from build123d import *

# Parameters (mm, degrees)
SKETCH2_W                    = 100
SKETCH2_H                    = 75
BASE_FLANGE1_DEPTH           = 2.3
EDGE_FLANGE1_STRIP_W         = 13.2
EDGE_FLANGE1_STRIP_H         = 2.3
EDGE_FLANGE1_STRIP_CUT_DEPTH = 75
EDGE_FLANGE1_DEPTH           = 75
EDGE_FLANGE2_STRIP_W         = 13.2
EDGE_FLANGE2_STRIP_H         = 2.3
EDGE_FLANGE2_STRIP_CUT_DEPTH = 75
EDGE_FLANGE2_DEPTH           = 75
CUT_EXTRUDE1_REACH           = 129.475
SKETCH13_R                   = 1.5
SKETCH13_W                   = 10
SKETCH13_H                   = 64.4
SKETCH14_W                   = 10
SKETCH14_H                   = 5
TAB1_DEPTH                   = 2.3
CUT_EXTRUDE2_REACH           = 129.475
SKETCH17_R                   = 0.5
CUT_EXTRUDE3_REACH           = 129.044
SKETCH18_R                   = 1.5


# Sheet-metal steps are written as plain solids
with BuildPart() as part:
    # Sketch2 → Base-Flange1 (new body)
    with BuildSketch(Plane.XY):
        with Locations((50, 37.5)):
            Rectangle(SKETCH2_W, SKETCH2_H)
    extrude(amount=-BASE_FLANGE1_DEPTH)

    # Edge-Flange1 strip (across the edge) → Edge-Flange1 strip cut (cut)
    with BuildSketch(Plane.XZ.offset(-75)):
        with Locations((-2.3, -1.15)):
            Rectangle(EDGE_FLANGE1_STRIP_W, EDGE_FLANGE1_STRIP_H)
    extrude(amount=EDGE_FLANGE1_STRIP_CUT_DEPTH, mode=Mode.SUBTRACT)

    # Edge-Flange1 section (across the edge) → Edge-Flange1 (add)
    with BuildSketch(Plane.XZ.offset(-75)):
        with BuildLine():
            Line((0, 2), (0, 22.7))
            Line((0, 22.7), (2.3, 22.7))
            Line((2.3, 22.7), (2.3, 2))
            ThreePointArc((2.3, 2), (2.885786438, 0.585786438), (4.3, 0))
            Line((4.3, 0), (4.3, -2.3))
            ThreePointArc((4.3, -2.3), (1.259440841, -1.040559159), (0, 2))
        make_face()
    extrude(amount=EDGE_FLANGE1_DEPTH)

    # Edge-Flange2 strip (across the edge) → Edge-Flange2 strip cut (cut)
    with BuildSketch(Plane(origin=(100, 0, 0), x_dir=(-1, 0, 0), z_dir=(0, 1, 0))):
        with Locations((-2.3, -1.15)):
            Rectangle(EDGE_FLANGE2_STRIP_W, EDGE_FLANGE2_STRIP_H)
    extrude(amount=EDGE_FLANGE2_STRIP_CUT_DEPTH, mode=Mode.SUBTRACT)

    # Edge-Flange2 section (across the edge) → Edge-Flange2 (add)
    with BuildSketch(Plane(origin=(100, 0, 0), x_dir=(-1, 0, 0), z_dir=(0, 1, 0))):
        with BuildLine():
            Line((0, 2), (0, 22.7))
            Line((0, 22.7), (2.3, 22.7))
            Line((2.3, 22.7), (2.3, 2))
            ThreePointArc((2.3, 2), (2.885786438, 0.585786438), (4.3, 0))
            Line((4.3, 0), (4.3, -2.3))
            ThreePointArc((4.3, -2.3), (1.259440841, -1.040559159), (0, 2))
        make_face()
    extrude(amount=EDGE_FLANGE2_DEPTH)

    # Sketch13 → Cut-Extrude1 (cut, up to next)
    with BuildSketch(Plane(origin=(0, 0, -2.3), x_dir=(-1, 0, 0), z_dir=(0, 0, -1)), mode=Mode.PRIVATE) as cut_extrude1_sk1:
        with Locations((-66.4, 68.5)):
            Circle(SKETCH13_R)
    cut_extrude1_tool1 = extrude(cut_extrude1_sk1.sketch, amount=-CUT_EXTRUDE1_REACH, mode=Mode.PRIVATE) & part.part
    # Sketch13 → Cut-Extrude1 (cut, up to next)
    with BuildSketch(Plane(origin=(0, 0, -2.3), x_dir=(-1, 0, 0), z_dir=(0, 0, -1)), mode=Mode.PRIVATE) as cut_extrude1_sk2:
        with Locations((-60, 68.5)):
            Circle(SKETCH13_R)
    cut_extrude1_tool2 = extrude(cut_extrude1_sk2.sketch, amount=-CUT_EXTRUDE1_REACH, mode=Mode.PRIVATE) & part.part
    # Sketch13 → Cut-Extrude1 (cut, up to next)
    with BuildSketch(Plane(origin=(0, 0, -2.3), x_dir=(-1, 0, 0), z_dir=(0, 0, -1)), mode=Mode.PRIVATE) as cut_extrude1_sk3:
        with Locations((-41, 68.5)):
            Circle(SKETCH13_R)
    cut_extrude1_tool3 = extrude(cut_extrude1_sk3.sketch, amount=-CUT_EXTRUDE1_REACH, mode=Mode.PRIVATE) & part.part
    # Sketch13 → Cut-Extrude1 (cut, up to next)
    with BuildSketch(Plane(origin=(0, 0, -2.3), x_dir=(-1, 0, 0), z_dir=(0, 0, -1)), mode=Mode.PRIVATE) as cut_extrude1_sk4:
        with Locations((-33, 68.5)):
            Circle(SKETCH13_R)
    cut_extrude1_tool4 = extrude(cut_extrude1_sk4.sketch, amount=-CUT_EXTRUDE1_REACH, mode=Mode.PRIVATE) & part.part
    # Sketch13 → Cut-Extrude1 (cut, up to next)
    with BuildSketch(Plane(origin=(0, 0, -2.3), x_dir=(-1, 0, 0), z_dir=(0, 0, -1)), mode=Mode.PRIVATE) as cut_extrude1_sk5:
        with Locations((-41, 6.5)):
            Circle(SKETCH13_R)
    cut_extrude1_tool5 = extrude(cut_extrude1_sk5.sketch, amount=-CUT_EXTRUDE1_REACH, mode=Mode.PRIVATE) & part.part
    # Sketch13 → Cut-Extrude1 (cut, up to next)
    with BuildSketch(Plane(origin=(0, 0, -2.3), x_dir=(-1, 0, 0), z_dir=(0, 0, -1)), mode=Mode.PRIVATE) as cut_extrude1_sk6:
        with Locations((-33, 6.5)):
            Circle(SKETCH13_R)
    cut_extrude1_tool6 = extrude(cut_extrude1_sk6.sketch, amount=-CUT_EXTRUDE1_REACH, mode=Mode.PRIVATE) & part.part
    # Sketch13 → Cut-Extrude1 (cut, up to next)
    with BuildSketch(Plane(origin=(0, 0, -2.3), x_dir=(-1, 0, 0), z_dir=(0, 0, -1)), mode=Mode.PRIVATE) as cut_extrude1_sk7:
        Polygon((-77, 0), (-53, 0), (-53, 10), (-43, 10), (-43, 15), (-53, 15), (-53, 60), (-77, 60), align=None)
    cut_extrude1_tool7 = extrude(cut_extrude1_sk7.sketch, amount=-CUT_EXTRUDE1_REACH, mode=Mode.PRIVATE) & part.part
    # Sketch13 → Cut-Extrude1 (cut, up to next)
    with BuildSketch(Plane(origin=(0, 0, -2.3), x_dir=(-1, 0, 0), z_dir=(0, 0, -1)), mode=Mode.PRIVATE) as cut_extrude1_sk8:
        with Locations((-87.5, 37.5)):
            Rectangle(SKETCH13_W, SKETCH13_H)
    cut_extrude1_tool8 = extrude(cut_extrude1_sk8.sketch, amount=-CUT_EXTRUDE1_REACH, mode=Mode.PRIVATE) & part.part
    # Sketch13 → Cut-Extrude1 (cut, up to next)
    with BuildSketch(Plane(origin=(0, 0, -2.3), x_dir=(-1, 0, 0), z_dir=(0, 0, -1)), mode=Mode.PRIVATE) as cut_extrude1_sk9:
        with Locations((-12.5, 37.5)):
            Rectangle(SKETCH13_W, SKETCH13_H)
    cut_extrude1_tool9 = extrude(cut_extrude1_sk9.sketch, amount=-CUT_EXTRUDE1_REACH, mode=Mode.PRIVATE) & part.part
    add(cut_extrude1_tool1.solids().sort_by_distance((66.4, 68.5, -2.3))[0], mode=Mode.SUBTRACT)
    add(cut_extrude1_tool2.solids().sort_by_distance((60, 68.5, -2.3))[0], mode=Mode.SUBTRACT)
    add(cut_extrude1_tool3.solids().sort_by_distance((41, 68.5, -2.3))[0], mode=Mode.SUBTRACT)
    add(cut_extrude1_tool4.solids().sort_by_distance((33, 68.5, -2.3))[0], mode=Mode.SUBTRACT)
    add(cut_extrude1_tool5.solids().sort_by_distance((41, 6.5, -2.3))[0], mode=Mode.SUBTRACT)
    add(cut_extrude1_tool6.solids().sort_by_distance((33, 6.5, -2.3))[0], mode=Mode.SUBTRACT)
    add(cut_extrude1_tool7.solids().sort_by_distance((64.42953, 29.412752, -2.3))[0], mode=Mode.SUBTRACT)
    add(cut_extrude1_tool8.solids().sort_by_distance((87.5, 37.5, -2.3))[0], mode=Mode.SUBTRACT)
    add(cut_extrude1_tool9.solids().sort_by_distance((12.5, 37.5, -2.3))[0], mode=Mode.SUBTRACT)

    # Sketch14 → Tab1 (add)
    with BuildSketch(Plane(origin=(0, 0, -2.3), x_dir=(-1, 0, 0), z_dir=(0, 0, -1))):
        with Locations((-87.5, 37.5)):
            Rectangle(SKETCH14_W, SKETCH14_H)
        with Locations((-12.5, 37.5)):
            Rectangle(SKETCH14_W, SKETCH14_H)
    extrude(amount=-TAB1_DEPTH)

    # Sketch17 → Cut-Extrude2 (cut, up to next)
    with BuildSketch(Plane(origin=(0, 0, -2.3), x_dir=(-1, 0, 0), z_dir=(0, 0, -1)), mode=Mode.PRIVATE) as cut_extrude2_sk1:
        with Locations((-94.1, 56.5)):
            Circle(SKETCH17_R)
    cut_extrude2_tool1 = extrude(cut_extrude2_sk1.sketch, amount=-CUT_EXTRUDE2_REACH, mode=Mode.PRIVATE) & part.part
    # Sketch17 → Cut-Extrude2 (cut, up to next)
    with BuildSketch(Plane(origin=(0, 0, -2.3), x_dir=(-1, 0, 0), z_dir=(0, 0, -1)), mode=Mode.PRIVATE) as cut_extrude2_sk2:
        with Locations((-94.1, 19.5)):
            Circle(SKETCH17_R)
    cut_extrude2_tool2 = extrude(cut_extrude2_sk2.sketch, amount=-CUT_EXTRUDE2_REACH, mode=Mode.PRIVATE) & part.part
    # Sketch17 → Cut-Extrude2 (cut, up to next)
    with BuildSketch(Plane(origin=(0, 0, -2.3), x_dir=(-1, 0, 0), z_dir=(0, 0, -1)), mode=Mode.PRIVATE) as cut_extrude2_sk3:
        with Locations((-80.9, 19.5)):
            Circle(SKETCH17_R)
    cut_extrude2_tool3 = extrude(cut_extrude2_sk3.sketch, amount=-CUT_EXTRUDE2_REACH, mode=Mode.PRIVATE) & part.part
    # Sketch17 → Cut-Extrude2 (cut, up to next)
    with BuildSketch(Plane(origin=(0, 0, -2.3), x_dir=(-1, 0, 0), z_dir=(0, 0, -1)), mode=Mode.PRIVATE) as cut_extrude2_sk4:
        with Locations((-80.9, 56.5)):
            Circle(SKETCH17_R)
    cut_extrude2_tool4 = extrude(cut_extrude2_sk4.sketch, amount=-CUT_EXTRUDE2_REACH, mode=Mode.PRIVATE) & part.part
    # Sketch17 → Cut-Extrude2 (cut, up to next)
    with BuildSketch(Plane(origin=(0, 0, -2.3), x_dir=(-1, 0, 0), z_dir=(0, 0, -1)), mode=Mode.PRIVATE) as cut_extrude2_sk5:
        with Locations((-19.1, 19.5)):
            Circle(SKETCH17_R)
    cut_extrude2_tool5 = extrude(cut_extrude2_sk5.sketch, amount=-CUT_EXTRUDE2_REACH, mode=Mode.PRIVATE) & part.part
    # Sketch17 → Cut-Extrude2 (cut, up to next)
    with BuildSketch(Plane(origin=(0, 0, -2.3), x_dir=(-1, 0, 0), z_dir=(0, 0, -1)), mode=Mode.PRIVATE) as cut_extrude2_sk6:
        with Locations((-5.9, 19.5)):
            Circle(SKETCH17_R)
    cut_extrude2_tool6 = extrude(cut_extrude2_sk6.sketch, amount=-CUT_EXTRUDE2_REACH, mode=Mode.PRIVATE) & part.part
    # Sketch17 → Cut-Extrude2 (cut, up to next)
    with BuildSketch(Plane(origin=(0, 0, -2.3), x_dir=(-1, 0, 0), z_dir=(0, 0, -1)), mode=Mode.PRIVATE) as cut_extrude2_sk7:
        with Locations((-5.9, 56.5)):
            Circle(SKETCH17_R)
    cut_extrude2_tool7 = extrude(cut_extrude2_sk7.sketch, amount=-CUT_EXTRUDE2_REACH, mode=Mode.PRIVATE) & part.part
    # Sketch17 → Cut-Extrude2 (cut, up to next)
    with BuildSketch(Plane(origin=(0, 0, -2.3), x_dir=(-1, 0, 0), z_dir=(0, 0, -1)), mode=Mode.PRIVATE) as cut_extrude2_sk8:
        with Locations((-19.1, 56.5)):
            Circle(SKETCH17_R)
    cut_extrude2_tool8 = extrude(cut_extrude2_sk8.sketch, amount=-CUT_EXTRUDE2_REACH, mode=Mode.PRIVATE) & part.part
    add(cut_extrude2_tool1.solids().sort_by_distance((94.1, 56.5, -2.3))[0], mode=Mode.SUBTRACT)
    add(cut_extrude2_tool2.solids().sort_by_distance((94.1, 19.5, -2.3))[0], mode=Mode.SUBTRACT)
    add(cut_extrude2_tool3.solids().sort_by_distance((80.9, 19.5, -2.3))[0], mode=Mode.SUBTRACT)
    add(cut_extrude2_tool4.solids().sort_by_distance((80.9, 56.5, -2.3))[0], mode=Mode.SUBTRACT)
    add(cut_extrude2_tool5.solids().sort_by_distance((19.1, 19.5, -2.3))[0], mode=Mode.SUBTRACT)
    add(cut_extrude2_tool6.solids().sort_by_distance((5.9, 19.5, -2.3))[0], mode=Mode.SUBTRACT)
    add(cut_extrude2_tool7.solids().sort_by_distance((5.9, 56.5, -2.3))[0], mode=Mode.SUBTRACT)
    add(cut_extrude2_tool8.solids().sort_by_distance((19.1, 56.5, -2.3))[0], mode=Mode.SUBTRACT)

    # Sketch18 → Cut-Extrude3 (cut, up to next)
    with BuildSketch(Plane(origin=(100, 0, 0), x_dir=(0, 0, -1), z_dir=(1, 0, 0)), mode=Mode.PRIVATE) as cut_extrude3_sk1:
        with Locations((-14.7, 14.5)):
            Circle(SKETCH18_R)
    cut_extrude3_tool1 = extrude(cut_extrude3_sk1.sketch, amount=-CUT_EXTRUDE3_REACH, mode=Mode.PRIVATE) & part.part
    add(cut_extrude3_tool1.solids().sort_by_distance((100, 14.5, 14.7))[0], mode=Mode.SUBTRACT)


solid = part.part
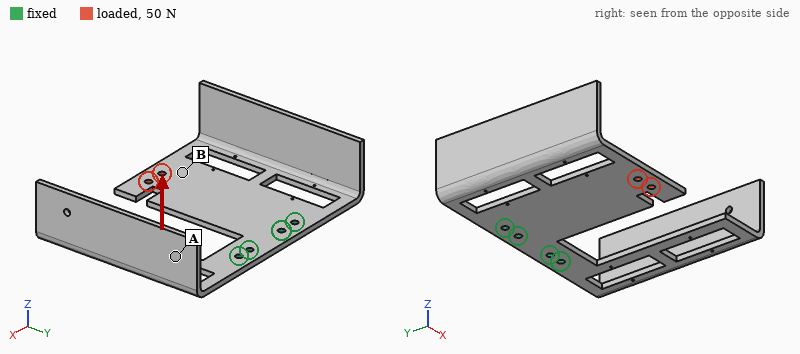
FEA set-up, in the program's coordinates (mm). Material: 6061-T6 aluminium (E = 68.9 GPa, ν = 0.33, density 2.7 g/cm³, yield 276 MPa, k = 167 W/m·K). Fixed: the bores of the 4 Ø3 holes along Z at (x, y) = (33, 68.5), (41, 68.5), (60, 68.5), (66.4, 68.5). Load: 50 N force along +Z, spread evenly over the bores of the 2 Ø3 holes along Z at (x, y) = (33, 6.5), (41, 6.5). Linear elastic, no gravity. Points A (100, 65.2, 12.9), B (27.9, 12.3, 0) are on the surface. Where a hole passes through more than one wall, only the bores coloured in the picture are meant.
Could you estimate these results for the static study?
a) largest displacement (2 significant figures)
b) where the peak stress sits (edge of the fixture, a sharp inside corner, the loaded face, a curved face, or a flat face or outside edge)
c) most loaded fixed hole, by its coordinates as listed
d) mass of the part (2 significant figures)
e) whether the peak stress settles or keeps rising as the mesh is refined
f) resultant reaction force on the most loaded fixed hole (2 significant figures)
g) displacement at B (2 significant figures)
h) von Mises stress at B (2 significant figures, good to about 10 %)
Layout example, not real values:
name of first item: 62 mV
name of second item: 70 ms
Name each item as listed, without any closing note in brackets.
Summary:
largest displacement: 1.4 mm
where the peak stress sits: edge of the fixture
most loaded fixed hole, by its coordinates as listed: (41, 68.5)
mass of the part: 49 g
whether the peak stress settles or keeps rising as the mesh is refined: keeps rising
resultant reaction force on the most loaded fixed hole: 48 N
displacement at B: 1.0 mm
von Mises stress at B: 23 MPa
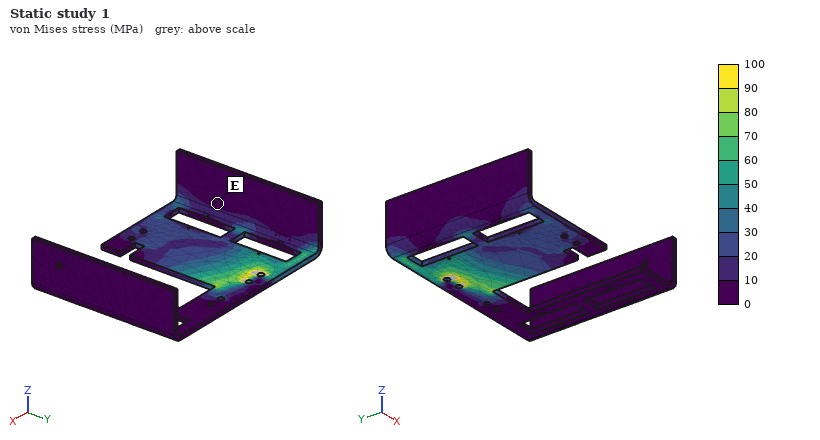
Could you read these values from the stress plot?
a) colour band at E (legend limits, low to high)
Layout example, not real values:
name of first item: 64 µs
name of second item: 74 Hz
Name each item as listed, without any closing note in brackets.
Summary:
colour band at E: 0 to 10 MPa
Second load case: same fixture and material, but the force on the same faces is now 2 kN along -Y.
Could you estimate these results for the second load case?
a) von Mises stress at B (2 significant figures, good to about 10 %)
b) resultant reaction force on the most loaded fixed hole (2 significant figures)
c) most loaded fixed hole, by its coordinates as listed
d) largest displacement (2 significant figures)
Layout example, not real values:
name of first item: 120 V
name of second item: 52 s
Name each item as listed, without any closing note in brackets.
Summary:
von Mises stress at B: 21 MPa
resultant reaction force on the most loaded fixed hole: 1.2 kN
most loaded fixed hole, by its coordinates as listed: (33, 68.5)
largest displacement: 45 µm
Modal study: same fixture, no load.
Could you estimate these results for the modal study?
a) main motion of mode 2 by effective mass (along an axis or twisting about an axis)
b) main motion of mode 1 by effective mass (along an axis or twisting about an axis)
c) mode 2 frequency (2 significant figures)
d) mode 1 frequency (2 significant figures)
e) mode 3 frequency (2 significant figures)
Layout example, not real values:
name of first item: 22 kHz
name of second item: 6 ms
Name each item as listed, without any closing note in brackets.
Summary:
main motion of mode 2 by effective mass: along Z
main motion of mode 1 by effective mass: along Z
mode 2 frequency: 280 Hz
mode 1 frequency: 190 Hz
mode 3 frequency: 440 Hz
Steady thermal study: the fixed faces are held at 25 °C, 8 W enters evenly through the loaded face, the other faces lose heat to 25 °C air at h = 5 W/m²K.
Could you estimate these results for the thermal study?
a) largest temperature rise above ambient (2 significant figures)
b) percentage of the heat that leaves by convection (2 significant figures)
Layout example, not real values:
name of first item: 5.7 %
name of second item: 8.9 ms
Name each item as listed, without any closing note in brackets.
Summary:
largest temperature rise above ambient: 39 K
percentage of the heat that leaves by convection: 11 %
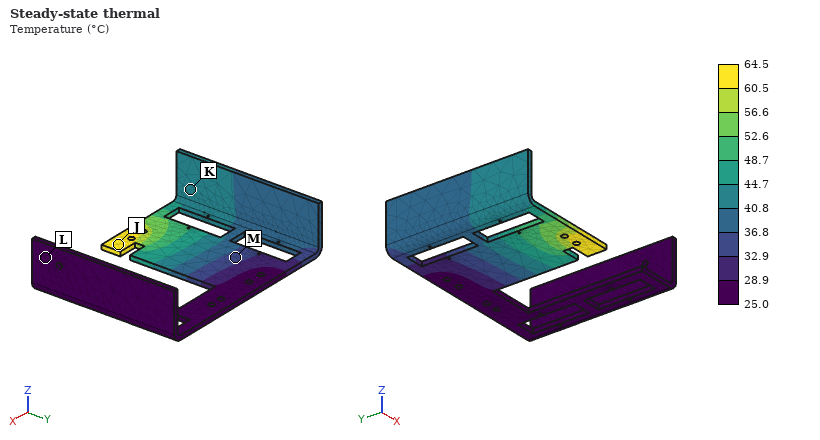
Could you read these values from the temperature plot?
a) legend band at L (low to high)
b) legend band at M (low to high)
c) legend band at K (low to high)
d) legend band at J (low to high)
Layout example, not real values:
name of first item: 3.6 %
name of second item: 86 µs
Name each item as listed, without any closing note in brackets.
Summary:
legend band at L: 25.0 to 28.9 °C
legend band at M: 32.9 to 36.8 °C
legend band at K: 40.8 to 44.7 °C
legend band at J: 60.5 to 64.5 °C
